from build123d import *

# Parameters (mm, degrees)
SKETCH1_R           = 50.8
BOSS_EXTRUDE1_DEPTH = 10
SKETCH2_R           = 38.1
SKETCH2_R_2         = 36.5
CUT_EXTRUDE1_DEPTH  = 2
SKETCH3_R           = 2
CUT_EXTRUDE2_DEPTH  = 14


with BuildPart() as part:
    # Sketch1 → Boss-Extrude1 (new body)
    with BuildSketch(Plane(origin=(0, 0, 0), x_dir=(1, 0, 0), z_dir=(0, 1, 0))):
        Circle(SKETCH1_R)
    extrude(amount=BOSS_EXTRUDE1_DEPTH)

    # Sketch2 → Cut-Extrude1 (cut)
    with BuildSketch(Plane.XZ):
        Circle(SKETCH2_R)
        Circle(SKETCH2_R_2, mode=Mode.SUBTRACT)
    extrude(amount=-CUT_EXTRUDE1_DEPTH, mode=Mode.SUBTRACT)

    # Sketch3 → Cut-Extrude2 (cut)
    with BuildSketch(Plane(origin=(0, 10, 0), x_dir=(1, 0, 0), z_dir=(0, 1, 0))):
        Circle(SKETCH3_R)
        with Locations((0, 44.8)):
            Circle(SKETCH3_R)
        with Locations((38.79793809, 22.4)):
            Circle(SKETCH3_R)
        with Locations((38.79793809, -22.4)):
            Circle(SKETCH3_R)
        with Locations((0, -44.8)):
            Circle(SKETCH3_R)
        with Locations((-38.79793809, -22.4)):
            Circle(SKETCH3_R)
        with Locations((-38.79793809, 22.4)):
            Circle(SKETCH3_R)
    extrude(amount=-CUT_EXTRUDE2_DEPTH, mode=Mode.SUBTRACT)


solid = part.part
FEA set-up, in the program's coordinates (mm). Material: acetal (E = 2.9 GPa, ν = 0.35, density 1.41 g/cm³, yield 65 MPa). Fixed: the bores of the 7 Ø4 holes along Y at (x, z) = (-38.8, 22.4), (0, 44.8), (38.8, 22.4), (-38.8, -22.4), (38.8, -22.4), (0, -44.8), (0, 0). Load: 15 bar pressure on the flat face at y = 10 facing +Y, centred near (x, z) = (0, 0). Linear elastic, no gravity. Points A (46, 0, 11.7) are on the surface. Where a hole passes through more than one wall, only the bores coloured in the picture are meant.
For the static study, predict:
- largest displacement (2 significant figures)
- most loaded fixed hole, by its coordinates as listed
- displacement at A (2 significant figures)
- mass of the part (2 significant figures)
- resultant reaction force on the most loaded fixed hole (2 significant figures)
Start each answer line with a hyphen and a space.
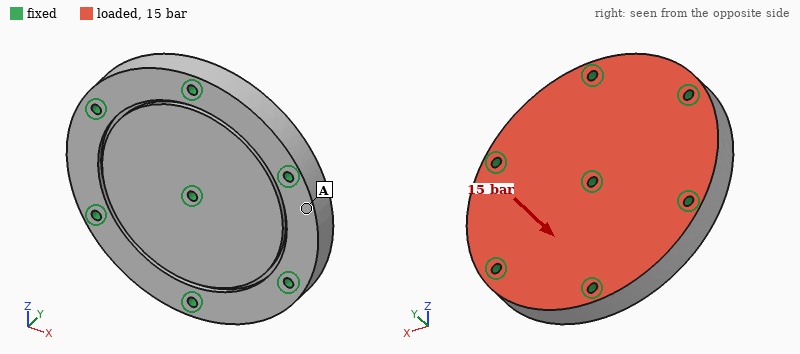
- 0.16 mm
- (0, 0)
- 0.088 mm
- 110 g
- 2.8 kN
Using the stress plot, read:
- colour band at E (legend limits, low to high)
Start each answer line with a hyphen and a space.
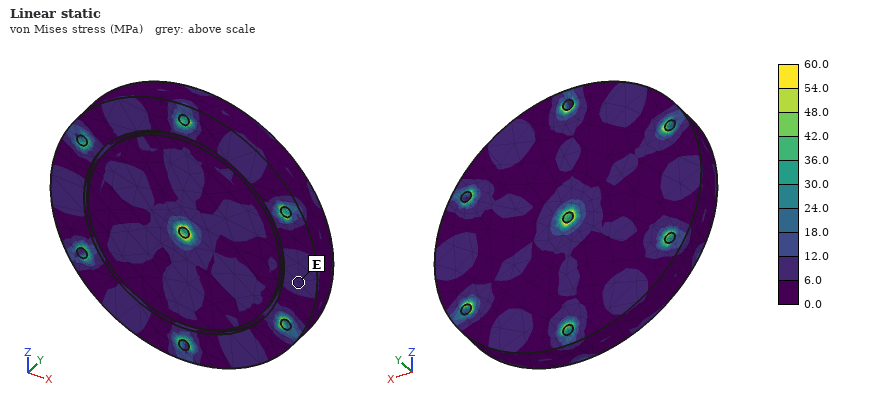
- 6.0 to 12.0 MPa
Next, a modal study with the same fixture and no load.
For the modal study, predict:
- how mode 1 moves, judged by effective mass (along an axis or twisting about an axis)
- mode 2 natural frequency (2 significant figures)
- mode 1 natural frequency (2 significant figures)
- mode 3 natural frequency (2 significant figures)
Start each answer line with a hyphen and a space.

- along Y
- 4800 Hz
- 4600 Hz
- 4800 Hz
